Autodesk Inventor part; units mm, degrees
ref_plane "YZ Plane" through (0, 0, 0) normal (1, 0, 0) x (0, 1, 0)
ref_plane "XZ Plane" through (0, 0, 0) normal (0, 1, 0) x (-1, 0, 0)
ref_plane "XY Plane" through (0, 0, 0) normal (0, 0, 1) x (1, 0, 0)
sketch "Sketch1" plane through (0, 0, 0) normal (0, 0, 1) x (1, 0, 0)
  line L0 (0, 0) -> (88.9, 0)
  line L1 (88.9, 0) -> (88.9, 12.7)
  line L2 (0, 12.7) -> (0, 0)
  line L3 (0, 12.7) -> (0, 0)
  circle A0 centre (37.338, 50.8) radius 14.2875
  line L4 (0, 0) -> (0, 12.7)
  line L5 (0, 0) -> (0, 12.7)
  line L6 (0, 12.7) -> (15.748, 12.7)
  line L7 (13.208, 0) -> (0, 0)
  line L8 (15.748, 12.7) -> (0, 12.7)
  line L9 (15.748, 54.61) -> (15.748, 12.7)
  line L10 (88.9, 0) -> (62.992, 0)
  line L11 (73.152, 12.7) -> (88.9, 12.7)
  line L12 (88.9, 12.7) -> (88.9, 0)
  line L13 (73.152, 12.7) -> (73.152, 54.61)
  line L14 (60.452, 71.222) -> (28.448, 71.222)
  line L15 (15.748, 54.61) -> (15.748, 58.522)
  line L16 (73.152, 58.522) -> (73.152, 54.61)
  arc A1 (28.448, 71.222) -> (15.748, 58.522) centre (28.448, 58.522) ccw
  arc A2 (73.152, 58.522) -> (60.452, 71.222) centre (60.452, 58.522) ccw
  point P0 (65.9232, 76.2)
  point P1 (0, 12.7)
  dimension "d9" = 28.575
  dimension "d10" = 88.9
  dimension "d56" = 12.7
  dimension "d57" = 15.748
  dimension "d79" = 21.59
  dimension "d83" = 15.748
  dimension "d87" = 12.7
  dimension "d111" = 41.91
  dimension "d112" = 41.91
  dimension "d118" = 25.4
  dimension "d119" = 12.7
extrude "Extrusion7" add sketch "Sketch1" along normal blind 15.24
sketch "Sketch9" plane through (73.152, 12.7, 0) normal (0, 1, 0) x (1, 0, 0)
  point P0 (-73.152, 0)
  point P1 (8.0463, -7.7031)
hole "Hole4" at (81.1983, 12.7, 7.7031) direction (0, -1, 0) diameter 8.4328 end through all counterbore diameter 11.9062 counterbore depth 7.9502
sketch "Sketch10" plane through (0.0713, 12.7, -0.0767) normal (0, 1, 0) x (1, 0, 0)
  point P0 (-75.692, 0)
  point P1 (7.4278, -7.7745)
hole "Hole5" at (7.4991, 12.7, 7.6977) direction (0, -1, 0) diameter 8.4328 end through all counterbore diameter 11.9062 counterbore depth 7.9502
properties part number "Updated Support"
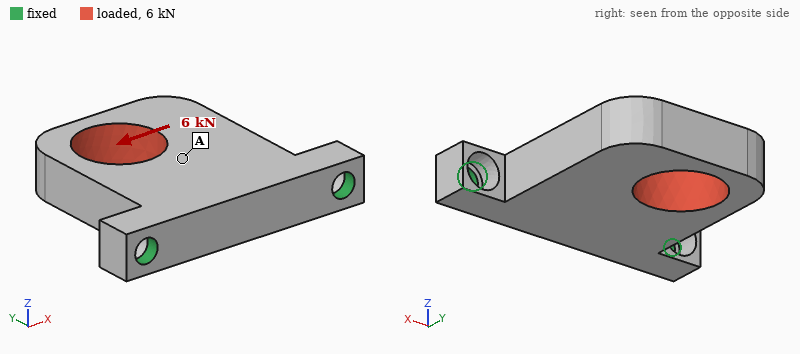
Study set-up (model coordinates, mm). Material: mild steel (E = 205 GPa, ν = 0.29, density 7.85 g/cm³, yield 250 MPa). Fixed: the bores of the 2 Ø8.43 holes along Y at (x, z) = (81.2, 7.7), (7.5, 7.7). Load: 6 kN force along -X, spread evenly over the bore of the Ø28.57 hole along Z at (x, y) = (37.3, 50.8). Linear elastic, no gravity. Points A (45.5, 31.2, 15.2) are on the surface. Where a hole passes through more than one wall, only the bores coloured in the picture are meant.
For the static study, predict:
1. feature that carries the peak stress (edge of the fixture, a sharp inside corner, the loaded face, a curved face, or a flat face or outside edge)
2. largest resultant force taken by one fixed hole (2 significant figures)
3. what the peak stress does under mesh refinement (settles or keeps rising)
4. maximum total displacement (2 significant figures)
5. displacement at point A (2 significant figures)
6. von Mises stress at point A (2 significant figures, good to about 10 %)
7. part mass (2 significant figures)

edge of the fixture
5.4 kN
keeps rising
30 µm
8.3 µm
25 MPa
430 g
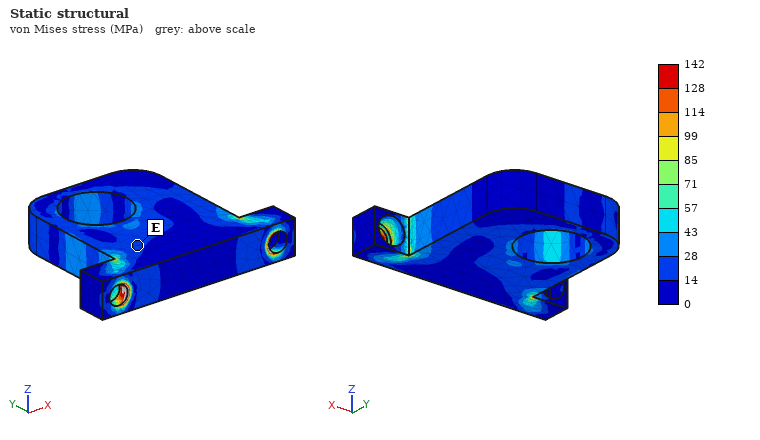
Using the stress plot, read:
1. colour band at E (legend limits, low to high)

14 to 28 MPa
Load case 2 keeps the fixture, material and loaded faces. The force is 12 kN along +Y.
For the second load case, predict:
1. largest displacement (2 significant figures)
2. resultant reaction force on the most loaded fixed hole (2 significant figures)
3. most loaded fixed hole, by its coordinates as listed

25 µm
8.2 kN
(7.5, 7.7)
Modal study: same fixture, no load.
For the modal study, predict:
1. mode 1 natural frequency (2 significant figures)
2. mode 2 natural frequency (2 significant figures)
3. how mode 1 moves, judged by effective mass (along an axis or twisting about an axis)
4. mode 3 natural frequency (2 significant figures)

1300 Hz
5500 Hz
along Z
5600 Hz
